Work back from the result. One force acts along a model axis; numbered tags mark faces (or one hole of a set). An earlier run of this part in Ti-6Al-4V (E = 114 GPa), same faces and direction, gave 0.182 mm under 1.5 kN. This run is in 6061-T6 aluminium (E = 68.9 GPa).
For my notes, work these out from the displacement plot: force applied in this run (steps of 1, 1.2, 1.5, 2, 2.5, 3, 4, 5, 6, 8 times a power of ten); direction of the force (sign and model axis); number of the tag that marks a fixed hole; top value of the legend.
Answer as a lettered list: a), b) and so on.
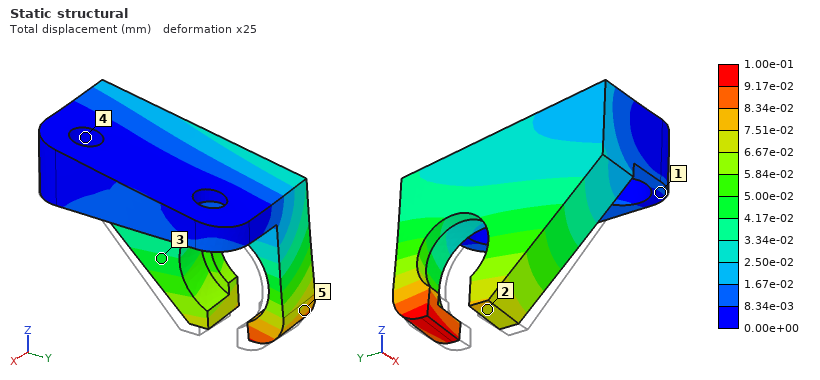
a) 500 N
b) -X
c) 4
d) 1.00e-01 mm
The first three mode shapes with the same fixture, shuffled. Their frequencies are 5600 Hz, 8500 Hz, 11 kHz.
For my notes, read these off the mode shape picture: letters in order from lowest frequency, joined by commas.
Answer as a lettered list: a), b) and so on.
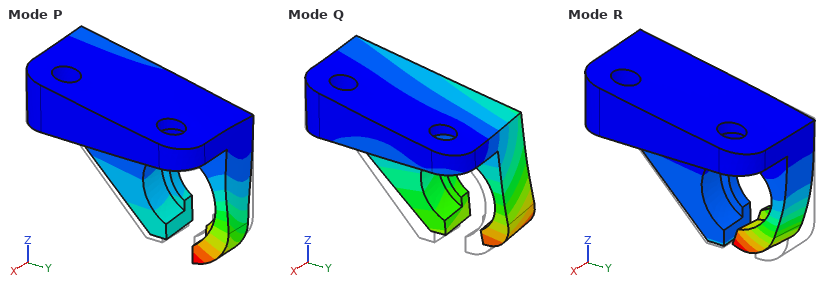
a) Q, R, P
